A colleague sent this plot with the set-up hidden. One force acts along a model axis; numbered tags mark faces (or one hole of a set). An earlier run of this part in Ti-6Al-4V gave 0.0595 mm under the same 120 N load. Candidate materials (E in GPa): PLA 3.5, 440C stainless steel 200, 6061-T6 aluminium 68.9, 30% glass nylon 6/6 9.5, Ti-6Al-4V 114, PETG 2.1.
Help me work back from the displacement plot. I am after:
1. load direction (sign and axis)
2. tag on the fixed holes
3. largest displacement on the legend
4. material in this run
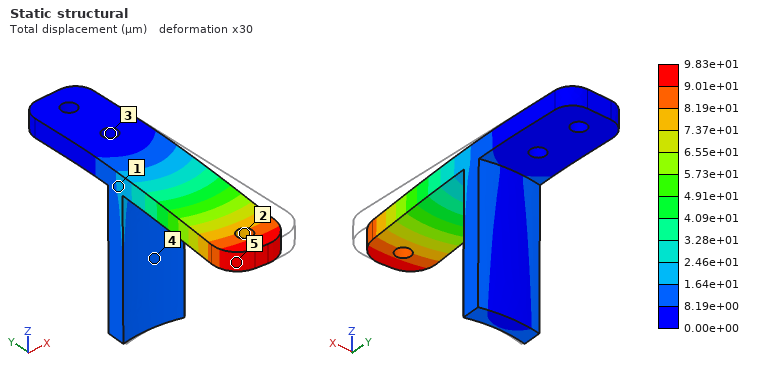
-X
3
9.83e+01 µm
6061-T6 aluminium
